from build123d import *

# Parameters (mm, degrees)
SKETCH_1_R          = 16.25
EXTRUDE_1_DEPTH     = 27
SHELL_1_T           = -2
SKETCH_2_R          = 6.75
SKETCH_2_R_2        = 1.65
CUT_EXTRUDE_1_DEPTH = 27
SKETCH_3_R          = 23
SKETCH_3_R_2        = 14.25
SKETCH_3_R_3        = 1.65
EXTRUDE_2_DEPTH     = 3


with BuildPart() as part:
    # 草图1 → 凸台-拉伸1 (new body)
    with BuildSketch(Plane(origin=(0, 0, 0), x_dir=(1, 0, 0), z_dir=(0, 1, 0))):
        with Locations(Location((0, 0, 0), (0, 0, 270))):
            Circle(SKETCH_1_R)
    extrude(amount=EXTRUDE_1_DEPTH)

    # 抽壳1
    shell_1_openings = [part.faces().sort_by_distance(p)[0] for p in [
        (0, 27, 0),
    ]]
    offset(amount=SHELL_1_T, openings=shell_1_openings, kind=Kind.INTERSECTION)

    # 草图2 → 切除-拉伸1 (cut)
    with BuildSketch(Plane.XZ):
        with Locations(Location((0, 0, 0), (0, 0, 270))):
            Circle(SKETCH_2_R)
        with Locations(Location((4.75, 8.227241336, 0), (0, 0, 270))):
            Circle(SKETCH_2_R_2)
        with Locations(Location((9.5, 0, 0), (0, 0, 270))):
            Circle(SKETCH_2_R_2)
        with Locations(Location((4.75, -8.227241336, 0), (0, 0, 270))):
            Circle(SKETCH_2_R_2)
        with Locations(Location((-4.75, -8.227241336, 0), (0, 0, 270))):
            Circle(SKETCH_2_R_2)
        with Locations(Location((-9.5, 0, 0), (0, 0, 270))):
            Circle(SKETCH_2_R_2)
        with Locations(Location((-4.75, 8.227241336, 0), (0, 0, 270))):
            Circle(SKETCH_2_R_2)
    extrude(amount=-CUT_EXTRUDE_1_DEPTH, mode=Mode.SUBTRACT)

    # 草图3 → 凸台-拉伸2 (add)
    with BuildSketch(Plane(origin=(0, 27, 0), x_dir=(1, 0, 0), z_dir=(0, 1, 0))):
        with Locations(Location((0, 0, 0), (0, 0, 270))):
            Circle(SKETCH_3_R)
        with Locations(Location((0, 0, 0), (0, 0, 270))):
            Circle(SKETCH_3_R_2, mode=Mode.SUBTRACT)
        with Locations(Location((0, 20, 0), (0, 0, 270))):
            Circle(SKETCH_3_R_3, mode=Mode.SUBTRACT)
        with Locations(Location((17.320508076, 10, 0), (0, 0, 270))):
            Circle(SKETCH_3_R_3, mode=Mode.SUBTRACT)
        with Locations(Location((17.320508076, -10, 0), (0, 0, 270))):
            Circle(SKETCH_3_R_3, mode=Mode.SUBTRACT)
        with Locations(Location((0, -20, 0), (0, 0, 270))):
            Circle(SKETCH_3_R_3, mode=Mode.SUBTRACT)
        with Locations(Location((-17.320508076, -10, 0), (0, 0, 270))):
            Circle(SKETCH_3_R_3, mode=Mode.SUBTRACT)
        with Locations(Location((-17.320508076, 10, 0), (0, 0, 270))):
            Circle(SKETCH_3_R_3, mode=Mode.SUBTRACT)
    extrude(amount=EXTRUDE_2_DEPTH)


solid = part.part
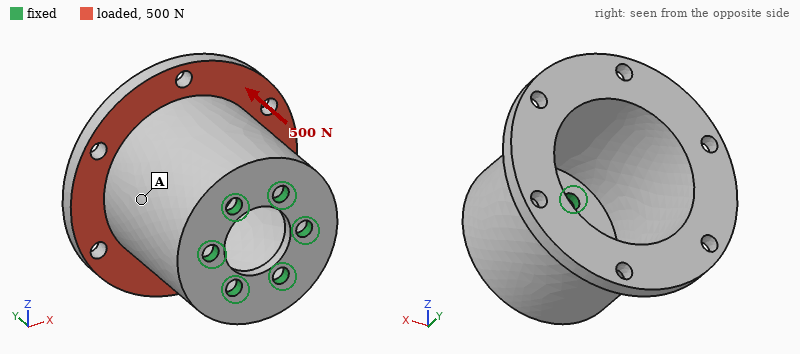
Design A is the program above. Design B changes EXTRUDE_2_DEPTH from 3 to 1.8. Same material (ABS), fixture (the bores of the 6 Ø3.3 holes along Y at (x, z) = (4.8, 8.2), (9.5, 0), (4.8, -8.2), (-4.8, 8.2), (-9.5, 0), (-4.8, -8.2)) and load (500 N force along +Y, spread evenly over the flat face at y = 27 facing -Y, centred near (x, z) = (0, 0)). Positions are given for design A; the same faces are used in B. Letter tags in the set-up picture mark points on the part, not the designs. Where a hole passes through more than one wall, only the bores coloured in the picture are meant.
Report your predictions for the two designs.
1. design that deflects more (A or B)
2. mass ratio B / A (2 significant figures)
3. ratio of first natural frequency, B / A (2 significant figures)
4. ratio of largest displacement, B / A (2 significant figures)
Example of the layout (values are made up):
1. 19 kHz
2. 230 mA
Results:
1. B
2. 0.87
3. 1.2
4. 1.7
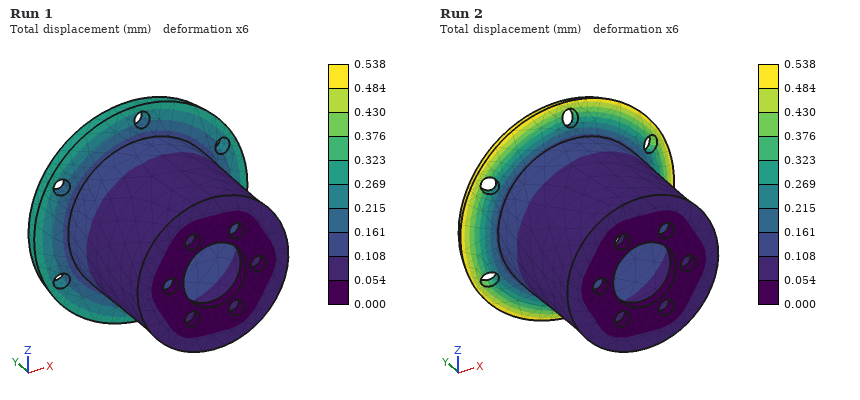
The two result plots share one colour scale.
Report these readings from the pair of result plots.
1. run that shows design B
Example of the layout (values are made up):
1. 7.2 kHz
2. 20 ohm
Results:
1. Run 2
